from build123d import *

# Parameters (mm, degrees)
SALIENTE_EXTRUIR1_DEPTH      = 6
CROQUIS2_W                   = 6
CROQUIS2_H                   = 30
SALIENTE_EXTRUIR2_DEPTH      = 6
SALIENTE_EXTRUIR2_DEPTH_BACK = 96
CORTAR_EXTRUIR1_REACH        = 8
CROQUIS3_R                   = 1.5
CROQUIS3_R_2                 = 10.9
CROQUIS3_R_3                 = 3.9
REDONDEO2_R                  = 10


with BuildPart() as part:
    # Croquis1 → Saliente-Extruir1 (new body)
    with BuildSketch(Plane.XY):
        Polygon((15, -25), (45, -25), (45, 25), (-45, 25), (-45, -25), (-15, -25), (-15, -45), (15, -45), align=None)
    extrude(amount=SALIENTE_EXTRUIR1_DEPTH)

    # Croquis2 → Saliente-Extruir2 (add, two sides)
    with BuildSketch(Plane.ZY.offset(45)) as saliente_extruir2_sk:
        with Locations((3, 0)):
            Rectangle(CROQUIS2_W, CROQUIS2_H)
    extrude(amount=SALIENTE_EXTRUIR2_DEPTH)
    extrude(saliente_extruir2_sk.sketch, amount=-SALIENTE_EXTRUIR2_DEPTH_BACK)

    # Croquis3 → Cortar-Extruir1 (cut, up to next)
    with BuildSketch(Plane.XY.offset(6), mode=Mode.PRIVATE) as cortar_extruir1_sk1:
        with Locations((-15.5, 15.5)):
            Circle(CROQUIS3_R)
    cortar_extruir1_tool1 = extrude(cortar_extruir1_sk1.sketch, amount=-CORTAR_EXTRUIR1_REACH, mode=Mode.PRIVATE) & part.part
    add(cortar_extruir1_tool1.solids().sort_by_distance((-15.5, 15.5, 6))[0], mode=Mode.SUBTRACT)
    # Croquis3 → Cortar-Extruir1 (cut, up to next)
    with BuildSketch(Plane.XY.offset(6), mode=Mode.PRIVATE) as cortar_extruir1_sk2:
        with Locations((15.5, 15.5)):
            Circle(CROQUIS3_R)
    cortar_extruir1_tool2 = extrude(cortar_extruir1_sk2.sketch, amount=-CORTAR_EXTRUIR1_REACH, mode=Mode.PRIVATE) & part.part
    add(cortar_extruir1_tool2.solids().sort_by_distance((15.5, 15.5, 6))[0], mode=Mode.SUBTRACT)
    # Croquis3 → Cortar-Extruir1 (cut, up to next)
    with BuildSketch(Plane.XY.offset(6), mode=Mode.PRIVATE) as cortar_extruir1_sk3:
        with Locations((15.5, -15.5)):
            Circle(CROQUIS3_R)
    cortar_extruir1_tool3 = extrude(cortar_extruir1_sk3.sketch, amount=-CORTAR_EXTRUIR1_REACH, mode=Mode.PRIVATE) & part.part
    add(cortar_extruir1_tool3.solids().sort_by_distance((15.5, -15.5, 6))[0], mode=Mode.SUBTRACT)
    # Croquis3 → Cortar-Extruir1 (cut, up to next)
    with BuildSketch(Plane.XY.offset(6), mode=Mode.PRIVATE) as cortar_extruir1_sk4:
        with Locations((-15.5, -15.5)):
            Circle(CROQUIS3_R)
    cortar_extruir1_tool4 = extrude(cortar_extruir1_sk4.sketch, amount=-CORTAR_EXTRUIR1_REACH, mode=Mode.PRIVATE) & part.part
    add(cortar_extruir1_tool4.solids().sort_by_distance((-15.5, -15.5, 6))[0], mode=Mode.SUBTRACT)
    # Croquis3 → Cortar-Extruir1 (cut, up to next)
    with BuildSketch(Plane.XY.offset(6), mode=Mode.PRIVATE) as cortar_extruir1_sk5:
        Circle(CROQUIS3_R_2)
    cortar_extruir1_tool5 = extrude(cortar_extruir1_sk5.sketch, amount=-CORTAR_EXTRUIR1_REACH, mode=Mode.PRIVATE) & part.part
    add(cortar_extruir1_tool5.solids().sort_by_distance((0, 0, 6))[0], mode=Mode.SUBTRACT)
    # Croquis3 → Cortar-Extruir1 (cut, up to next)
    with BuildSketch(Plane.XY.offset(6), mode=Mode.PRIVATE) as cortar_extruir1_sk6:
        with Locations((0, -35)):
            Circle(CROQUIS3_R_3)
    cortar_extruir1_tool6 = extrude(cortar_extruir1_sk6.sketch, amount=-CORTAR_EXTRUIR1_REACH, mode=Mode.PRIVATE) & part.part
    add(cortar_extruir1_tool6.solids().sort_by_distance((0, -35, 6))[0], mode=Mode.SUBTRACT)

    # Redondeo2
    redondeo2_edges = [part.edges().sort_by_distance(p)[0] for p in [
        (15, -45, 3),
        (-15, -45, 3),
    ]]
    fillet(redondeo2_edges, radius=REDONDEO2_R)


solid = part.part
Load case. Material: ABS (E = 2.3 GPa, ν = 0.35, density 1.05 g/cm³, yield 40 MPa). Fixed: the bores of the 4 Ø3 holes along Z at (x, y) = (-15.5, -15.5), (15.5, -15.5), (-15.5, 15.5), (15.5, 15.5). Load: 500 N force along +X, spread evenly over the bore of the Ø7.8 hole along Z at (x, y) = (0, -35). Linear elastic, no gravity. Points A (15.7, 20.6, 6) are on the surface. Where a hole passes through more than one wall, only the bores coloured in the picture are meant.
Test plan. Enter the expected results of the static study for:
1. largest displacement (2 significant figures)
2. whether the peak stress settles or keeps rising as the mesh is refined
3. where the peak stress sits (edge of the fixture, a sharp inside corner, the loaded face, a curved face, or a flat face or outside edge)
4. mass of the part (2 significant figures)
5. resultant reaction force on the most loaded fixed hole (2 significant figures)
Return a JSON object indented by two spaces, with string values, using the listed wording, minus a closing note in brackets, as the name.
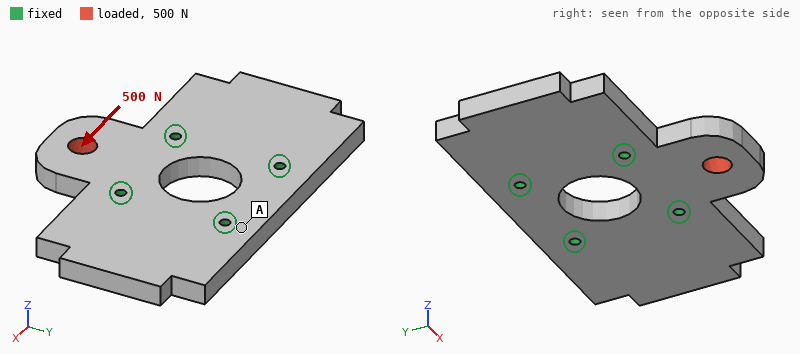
{
  "largest displacement": "0.12 mm",
  "whether the peak stress settles or keeps rising as the mesh is refined": "keeps rising",
  "where the peak stress sits": "edge of the fixture",
  "mass of the part": "31 g",
  "resultant reaction force on the most loaded fixed hole": "360 N"
}
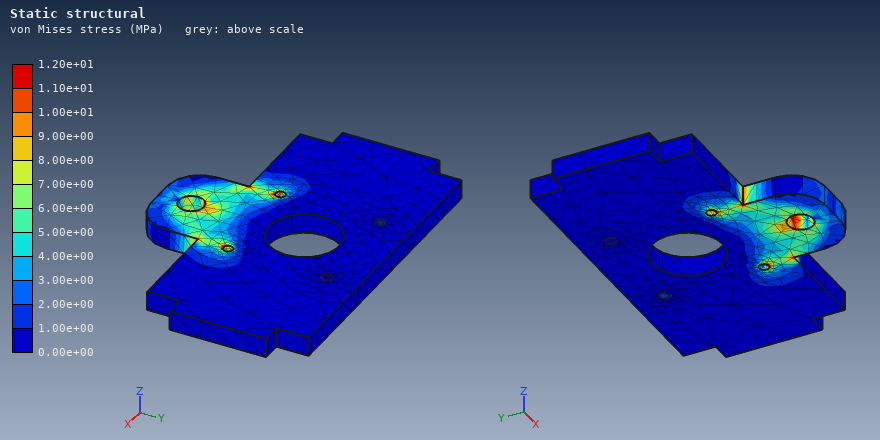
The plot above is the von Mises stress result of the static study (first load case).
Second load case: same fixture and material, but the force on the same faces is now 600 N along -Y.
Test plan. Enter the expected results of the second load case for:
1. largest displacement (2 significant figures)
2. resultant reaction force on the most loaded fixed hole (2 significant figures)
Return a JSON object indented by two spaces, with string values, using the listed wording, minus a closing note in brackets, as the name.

{
  "largest displacement": "68 µm",
  "resultant reaction force on the most loaded fixed hole": "290 N"
}
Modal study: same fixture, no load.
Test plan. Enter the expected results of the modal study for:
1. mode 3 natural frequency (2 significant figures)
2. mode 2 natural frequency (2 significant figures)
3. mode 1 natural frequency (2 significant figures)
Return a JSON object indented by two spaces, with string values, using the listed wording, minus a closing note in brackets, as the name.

{
  "mode 3 natural frequency": "1700 Hz",
  "mode 2 natural frequency": "1100 Hz",
  "mode 1 natural frequency": "1100 Hz"
}
